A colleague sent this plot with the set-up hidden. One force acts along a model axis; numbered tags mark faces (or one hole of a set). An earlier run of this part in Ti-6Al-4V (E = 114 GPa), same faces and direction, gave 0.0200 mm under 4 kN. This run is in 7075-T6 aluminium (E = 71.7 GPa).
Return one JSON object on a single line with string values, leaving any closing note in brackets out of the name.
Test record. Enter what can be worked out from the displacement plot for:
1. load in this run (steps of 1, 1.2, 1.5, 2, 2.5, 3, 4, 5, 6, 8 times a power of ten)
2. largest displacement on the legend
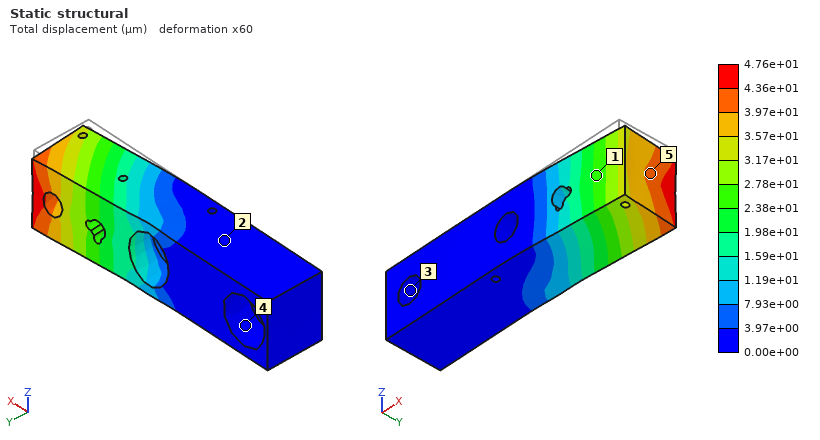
{"load in this run": "6 kN", "largest displacement on the legend": "4.76e+01 µm"}
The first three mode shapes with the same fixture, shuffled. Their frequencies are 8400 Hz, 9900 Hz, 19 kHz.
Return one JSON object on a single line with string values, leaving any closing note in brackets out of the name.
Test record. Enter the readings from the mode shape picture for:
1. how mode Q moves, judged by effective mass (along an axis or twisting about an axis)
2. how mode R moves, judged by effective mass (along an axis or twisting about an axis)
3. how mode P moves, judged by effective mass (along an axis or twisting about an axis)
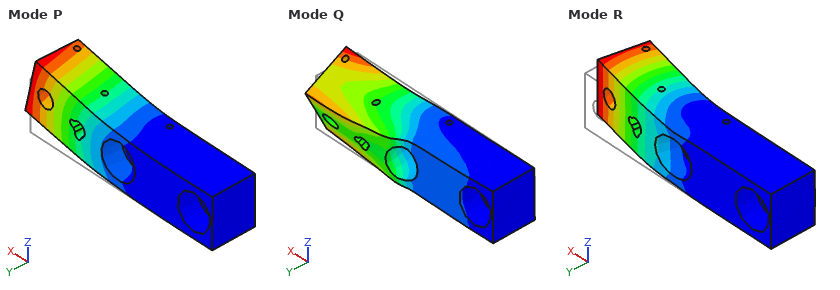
{"how mode Q moves, judged by effective mass": "twisting about X", "how mode R moves, judged by effective mass": "along Y", "how mode P moves, judged by effective mass": "along Z"}
